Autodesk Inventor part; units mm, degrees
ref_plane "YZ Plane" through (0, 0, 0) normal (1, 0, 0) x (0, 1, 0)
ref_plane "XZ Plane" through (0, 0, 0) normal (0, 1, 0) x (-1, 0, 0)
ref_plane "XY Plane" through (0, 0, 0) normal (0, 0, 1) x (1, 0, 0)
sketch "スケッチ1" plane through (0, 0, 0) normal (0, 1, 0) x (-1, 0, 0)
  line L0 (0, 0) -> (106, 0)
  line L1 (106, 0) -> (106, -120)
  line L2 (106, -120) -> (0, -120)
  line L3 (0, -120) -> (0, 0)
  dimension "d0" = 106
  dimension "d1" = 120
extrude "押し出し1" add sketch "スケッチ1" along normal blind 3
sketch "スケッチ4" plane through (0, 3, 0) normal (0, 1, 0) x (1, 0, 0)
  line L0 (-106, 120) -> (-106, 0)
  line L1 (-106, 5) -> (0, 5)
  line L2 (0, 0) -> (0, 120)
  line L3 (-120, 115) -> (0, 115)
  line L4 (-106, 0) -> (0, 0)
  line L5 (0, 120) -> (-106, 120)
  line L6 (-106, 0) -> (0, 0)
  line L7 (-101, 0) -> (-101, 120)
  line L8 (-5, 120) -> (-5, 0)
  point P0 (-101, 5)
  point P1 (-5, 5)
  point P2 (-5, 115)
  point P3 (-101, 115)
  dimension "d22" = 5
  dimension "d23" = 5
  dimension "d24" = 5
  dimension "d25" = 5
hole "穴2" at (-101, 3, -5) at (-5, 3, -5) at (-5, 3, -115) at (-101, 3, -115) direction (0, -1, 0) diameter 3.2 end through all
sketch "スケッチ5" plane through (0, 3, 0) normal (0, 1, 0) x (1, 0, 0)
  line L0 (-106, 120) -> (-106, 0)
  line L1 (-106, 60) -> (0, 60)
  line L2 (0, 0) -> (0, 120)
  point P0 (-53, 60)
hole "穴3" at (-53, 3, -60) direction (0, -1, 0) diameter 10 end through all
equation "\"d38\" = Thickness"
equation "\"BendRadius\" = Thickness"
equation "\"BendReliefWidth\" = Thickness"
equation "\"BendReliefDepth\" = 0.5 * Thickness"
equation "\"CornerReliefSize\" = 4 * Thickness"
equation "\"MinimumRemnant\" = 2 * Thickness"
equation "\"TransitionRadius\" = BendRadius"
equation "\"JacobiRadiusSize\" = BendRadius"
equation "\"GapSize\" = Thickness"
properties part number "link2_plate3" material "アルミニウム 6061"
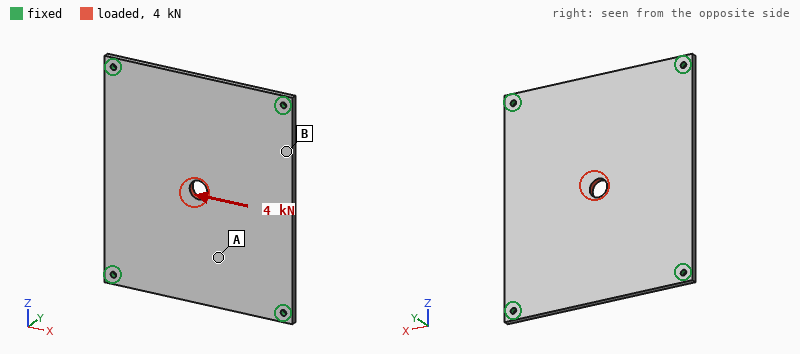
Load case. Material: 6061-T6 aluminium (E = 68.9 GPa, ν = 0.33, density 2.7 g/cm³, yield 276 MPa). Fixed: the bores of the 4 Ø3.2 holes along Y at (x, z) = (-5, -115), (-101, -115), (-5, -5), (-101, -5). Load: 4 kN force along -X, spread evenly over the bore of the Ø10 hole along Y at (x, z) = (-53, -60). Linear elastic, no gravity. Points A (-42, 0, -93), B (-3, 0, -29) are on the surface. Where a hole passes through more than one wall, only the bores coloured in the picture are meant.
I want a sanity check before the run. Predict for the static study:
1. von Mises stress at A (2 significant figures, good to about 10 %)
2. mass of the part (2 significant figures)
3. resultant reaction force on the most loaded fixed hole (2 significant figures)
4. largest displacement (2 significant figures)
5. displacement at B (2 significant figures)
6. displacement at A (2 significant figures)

12 MPa
100 g
1.2 kN
26 µm
13 µm
12 µm
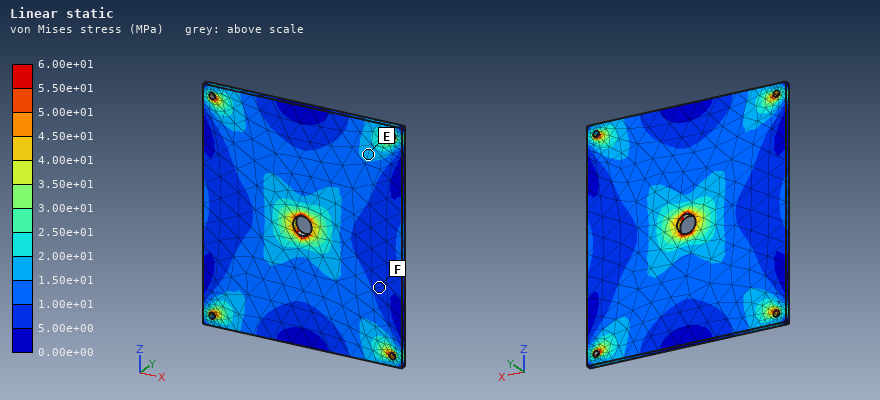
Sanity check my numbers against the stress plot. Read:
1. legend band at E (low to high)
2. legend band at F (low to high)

1.50e+01 to 2.00e+01 MPa
5.00e+00 to 1.00e+01 MPa
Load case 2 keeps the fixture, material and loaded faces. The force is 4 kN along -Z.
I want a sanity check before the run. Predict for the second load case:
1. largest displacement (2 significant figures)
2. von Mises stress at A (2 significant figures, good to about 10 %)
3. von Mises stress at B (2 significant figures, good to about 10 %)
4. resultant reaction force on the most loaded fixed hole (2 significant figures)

23 µm
9.0 MPa
10 MPa
1.1 kN
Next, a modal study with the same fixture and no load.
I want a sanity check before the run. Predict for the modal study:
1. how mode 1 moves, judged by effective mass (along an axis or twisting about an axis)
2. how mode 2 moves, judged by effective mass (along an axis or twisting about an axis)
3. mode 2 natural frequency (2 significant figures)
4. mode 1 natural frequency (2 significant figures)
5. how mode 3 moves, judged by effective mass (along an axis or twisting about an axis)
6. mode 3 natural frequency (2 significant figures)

along Y
twisting about Z
1500 Hz
850 Hz
twisting about X
1700 Hz
